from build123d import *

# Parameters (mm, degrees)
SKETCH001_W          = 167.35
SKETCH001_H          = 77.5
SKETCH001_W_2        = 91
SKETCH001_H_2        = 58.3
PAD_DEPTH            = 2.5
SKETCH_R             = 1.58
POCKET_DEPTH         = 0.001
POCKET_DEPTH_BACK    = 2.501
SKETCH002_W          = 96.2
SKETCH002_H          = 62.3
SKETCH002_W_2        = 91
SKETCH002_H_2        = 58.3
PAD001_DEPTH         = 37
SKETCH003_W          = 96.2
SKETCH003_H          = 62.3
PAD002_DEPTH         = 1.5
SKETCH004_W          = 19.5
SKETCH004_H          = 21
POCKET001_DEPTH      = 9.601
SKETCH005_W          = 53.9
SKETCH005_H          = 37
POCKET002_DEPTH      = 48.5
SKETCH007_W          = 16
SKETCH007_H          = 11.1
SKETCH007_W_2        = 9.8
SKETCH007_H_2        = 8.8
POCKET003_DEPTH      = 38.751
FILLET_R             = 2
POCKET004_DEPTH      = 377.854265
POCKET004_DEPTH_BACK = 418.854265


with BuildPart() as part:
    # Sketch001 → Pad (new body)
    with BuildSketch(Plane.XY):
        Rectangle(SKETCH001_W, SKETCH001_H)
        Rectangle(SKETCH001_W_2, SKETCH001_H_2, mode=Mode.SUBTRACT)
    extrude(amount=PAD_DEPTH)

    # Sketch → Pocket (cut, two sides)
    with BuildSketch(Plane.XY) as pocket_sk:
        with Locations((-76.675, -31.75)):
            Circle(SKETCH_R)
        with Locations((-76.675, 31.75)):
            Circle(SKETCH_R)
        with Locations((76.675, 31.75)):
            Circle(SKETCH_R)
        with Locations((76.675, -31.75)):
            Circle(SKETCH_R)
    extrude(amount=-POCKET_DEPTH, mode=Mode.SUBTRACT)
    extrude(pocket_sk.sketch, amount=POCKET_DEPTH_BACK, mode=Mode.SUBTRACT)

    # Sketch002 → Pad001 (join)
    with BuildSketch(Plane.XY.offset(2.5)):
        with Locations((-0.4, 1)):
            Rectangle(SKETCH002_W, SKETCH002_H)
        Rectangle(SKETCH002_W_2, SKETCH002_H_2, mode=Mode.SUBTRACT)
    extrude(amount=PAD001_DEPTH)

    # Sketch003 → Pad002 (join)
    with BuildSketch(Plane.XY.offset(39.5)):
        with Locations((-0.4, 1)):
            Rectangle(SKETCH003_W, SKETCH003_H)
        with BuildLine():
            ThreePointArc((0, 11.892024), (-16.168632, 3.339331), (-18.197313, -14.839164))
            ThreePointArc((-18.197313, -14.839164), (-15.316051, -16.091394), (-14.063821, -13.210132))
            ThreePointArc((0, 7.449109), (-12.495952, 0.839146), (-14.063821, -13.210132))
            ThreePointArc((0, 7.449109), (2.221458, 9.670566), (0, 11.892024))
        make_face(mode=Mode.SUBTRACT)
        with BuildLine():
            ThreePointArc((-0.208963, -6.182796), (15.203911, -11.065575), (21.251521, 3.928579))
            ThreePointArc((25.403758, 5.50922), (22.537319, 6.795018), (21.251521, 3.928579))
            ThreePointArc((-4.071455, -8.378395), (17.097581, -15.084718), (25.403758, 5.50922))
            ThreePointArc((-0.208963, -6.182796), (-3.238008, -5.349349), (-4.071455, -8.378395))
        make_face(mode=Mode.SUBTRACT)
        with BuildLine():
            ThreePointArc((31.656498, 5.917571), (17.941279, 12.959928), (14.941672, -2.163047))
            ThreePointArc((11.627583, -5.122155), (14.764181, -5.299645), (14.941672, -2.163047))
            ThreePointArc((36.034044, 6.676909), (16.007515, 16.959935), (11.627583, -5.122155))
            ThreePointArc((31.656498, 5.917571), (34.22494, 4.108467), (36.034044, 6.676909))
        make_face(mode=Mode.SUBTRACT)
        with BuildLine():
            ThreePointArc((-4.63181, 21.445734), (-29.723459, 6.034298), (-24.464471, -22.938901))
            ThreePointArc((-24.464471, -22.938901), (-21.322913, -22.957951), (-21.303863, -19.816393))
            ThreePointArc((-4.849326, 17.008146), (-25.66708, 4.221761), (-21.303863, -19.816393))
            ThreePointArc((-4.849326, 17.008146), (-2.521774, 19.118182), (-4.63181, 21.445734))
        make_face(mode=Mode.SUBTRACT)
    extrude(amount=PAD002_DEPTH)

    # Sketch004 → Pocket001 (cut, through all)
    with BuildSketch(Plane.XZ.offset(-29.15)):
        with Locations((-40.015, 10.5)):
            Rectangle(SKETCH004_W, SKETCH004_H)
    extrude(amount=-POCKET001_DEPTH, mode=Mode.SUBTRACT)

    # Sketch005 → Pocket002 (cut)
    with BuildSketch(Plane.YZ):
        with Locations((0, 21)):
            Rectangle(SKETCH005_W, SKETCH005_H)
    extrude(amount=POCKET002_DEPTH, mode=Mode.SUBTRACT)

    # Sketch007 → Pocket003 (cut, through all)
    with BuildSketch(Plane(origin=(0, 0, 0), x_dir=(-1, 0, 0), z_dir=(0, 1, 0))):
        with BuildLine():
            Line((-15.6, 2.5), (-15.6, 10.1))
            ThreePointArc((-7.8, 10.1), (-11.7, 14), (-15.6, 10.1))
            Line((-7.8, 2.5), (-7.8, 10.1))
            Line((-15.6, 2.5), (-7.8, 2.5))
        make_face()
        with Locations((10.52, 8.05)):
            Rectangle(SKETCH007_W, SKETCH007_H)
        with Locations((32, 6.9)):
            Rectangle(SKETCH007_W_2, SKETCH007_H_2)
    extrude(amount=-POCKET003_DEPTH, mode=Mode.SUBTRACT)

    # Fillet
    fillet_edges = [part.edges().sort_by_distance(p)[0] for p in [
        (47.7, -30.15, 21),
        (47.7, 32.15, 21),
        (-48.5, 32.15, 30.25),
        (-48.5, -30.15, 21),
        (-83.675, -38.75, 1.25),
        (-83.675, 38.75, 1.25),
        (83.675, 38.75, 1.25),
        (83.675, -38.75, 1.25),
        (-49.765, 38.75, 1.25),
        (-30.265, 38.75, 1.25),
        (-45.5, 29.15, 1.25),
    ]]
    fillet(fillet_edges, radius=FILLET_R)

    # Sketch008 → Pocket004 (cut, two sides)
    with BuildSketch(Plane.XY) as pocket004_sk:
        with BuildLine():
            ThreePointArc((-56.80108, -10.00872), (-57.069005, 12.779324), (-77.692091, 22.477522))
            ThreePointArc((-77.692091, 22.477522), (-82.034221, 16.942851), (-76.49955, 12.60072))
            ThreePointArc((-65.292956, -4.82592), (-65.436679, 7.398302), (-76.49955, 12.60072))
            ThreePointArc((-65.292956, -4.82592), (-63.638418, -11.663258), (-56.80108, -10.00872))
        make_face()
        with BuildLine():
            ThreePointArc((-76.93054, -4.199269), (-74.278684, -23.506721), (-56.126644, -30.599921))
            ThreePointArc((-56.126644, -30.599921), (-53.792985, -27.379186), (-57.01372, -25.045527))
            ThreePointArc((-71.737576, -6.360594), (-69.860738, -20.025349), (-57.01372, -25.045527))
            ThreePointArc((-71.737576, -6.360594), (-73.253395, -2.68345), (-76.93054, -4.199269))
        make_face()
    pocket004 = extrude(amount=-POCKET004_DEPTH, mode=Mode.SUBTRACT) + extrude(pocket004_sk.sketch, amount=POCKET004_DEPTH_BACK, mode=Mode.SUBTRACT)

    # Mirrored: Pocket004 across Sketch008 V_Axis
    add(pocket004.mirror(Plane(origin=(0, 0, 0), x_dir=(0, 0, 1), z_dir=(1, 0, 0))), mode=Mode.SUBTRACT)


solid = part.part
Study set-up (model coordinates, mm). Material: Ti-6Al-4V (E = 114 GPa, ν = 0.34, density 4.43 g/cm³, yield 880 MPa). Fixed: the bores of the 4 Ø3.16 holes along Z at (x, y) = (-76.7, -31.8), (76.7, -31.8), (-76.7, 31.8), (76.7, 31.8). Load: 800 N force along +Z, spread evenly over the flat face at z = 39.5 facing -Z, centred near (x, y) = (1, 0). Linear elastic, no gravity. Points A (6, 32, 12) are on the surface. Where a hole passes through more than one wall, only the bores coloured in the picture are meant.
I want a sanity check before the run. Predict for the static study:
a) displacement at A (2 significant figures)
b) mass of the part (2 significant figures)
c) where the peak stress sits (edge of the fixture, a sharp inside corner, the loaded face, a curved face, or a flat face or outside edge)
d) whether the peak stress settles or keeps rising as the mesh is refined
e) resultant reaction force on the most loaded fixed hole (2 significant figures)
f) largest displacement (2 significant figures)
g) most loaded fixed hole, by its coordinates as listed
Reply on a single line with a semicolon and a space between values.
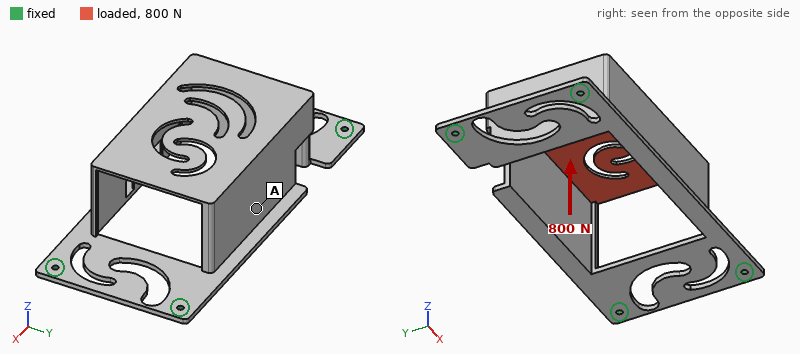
0.24 mm; 190 g; edge of the fixture; keeps rising; 300 N; 0.83 mm; (76.7, 31.8)
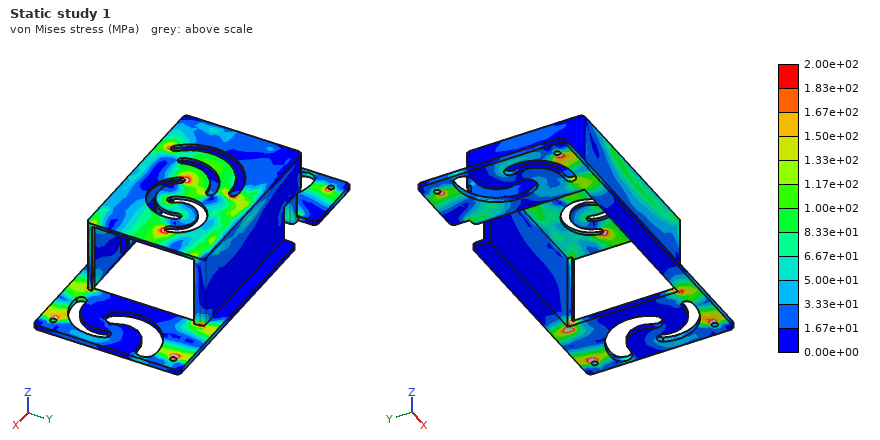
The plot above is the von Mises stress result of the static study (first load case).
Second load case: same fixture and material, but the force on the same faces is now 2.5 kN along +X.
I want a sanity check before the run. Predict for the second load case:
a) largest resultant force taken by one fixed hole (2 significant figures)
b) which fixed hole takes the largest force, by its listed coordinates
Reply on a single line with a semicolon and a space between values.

1.1 kN; (76.7, 31.8)
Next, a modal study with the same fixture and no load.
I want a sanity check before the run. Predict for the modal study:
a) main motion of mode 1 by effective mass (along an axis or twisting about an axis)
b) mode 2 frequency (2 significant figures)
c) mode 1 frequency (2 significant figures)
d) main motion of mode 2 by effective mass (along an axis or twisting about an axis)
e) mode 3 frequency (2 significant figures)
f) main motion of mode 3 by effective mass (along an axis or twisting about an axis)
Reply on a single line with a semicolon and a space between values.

along Y; 700 Hz; 560 Hz; along Z; 1000 Hz; along X
